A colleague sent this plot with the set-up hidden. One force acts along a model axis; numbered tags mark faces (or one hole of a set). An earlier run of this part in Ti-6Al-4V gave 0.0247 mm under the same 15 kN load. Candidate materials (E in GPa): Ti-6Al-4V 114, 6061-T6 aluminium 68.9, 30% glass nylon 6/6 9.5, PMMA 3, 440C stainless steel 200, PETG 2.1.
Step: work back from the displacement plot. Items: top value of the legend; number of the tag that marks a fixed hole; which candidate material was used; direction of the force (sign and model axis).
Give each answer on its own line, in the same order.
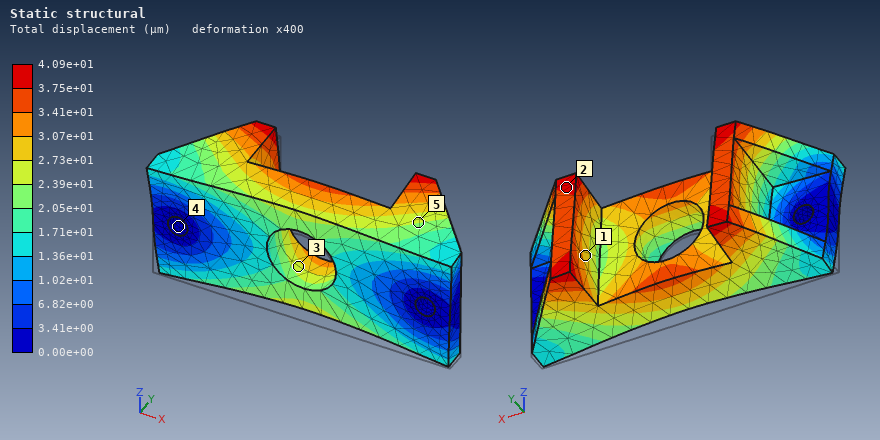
4.09e+01 µm
4
6061-T6 aluminium
+Z
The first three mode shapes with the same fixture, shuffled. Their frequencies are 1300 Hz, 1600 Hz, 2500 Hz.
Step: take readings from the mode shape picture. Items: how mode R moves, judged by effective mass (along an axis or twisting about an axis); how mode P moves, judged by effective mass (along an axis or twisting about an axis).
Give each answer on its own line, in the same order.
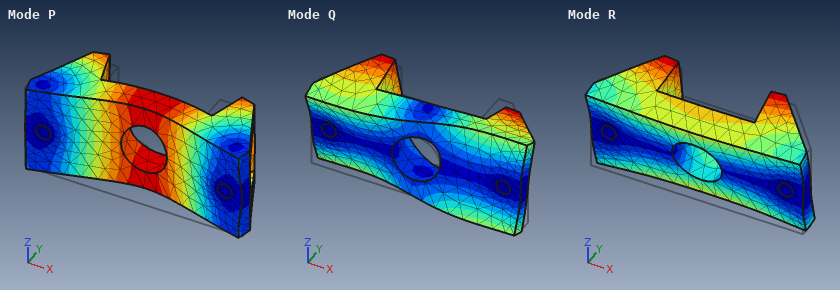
along Z
along Y
